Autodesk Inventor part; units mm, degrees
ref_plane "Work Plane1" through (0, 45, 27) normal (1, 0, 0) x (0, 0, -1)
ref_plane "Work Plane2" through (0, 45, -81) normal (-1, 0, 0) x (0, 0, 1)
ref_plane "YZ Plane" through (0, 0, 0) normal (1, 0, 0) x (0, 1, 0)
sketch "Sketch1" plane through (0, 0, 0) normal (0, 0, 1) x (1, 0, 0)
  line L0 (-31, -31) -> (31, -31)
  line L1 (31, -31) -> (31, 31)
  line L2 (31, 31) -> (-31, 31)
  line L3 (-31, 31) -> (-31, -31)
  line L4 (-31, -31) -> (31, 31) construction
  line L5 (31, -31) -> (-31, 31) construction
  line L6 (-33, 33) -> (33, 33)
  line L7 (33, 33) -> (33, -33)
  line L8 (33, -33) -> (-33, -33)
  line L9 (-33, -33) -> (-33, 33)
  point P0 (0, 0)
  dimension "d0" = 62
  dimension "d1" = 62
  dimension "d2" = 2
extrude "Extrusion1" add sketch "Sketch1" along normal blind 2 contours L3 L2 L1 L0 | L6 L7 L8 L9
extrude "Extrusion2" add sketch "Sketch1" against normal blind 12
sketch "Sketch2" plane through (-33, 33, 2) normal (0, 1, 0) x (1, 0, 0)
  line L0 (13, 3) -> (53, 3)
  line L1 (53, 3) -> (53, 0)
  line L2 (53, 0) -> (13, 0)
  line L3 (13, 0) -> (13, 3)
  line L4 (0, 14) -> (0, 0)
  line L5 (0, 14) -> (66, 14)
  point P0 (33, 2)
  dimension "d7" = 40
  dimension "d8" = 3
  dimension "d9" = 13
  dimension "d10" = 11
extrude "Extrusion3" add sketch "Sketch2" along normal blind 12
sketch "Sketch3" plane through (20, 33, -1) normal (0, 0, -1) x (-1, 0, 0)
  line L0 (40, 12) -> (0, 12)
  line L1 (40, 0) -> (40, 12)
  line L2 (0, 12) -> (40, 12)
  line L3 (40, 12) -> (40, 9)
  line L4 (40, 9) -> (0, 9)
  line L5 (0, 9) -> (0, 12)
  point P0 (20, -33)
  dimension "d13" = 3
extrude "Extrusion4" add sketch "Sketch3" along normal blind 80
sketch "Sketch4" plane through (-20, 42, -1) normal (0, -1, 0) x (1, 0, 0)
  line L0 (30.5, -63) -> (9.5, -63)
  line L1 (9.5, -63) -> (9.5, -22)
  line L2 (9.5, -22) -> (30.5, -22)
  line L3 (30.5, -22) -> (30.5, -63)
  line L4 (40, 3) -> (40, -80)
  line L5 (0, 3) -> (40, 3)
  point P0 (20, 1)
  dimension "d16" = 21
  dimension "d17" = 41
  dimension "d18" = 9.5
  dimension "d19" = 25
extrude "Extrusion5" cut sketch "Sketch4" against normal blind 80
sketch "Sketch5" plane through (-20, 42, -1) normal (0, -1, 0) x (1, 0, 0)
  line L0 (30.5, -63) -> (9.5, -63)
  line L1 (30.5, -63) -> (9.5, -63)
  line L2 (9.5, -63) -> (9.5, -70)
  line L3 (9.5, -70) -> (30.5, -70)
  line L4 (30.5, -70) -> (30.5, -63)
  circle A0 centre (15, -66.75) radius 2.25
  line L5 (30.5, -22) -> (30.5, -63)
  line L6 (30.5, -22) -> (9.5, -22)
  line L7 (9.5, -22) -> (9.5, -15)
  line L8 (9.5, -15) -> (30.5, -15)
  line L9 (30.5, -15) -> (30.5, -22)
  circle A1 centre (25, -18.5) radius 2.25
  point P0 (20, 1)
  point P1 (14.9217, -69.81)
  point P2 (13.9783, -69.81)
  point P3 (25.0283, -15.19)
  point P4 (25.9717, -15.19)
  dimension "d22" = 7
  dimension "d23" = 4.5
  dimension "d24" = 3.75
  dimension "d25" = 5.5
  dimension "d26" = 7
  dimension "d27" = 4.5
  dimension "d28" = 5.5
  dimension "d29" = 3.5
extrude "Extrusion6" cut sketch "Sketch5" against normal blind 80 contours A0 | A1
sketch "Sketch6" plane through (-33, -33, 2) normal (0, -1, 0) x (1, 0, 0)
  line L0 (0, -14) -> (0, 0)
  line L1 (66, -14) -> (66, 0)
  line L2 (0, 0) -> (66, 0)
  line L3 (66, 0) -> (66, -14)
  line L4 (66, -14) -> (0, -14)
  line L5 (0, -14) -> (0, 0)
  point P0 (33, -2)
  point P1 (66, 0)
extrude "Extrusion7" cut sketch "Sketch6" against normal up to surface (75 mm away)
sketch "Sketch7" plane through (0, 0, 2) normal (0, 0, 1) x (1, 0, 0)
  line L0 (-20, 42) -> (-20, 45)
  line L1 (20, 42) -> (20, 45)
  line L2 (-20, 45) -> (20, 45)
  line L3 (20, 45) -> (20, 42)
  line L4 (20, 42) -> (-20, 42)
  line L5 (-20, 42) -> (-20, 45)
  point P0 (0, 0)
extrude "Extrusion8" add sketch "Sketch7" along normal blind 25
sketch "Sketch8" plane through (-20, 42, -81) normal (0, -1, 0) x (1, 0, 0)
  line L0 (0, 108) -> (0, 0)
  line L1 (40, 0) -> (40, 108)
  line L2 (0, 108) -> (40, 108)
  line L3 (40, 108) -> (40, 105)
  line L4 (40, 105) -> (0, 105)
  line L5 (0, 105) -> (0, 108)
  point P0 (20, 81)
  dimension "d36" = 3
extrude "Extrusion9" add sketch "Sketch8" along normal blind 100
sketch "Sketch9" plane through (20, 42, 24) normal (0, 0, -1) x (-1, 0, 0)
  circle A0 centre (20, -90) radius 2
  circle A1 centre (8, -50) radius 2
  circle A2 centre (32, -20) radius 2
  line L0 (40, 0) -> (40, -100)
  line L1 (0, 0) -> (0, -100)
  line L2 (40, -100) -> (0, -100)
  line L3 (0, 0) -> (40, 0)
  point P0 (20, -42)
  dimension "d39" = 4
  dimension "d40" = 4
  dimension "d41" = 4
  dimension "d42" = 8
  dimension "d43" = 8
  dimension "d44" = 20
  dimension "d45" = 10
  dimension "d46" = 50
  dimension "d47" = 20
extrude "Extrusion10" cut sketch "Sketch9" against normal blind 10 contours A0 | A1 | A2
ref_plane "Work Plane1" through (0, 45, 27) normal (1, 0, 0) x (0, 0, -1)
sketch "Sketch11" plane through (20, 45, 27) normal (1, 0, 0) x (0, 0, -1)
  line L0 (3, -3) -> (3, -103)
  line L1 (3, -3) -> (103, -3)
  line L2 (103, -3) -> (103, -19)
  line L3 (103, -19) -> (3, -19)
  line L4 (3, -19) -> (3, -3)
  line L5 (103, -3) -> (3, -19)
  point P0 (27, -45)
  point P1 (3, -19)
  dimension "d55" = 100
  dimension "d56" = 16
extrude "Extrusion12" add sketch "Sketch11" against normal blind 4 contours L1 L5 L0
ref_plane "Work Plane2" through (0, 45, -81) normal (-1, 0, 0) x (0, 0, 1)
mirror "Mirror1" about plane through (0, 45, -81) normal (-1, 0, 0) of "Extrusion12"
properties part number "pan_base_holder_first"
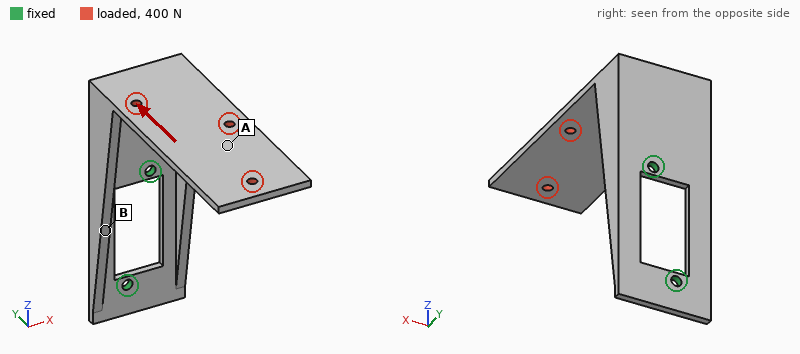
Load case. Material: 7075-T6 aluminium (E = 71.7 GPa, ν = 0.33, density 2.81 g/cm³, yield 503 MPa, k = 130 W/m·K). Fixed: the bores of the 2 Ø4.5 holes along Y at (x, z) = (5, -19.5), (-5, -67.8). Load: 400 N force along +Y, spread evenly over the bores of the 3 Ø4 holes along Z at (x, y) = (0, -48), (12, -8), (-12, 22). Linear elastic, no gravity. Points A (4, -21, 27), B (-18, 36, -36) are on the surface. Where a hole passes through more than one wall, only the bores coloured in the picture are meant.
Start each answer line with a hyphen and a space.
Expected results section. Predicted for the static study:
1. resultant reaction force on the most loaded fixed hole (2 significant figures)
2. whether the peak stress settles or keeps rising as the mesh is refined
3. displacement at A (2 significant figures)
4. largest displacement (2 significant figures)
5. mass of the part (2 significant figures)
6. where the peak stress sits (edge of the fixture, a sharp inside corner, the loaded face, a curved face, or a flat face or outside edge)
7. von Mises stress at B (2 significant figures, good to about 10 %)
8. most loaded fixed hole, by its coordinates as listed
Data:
- 750 N
- keeps rising
- 0.69 mm
- 1.0 mm
- 80 g
- edge of the fixture
- 56 MPa
- (5, -19.5)
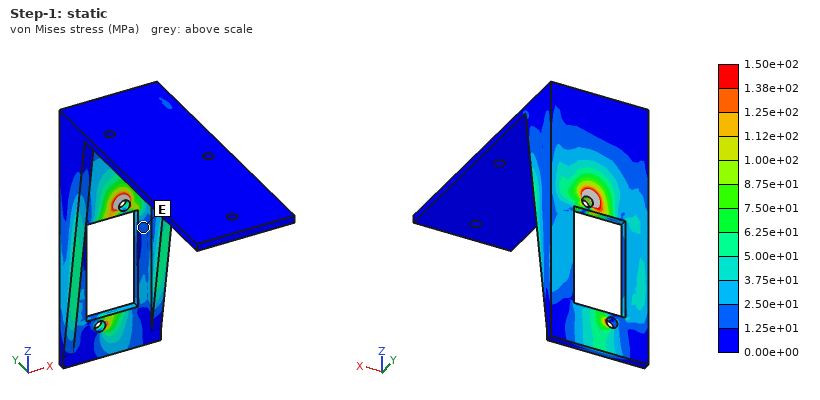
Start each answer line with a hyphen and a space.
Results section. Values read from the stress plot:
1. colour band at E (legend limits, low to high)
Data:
- 1.25e+01 to 2.50e+01 MPa
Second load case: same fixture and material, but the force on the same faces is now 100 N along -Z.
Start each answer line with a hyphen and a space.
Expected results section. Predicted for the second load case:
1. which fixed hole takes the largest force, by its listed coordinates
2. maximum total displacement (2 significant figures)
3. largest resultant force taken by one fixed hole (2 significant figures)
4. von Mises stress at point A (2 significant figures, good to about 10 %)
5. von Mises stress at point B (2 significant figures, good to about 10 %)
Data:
- (-5, -67.8)
- 1.6 mm
- 180 N
- 16 MPa
- 20 MPa
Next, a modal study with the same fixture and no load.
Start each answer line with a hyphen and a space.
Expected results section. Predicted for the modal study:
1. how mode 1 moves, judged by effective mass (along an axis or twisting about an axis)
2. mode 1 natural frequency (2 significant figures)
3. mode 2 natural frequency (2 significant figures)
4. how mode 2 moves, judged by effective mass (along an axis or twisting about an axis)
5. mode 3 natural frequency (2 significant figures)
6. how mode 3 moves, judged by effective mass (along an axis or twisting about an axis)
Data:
- along Z
- 280 Hz
- 300 Hz
- along X
- 840 Hz
- along Y
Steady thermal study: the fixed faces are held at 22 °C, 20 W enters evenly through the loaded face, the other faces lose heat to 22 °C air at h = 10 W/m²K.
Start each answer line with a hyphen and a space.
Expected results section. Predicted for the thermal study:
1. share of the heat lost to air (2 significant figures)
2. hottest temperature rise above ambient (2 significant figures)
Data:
- 33 %
- 79 K
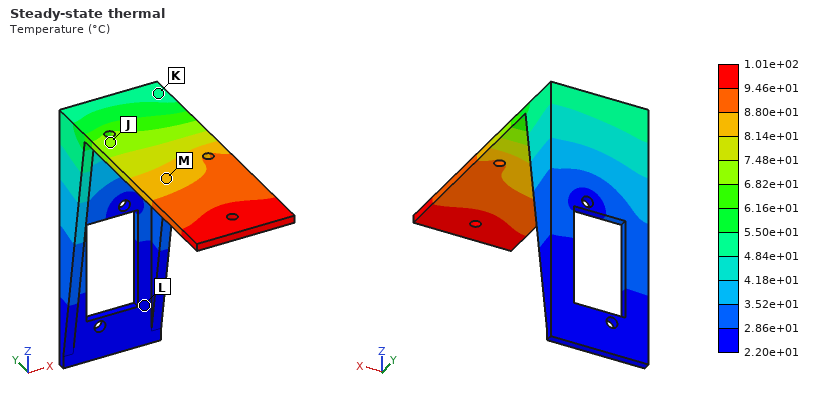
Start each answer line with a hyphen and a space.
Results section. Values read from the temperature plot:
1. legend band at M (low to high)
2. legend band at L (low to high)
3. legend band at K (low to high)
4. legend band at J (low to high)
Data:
- 8.14e+01 to 8.80e+01 °C
- 2.20e+01 to 2.86e+01 °C
- 4.84e+01 to 5.50e+01 °C
- 6.82e+01 to 7.48e+01 °C
